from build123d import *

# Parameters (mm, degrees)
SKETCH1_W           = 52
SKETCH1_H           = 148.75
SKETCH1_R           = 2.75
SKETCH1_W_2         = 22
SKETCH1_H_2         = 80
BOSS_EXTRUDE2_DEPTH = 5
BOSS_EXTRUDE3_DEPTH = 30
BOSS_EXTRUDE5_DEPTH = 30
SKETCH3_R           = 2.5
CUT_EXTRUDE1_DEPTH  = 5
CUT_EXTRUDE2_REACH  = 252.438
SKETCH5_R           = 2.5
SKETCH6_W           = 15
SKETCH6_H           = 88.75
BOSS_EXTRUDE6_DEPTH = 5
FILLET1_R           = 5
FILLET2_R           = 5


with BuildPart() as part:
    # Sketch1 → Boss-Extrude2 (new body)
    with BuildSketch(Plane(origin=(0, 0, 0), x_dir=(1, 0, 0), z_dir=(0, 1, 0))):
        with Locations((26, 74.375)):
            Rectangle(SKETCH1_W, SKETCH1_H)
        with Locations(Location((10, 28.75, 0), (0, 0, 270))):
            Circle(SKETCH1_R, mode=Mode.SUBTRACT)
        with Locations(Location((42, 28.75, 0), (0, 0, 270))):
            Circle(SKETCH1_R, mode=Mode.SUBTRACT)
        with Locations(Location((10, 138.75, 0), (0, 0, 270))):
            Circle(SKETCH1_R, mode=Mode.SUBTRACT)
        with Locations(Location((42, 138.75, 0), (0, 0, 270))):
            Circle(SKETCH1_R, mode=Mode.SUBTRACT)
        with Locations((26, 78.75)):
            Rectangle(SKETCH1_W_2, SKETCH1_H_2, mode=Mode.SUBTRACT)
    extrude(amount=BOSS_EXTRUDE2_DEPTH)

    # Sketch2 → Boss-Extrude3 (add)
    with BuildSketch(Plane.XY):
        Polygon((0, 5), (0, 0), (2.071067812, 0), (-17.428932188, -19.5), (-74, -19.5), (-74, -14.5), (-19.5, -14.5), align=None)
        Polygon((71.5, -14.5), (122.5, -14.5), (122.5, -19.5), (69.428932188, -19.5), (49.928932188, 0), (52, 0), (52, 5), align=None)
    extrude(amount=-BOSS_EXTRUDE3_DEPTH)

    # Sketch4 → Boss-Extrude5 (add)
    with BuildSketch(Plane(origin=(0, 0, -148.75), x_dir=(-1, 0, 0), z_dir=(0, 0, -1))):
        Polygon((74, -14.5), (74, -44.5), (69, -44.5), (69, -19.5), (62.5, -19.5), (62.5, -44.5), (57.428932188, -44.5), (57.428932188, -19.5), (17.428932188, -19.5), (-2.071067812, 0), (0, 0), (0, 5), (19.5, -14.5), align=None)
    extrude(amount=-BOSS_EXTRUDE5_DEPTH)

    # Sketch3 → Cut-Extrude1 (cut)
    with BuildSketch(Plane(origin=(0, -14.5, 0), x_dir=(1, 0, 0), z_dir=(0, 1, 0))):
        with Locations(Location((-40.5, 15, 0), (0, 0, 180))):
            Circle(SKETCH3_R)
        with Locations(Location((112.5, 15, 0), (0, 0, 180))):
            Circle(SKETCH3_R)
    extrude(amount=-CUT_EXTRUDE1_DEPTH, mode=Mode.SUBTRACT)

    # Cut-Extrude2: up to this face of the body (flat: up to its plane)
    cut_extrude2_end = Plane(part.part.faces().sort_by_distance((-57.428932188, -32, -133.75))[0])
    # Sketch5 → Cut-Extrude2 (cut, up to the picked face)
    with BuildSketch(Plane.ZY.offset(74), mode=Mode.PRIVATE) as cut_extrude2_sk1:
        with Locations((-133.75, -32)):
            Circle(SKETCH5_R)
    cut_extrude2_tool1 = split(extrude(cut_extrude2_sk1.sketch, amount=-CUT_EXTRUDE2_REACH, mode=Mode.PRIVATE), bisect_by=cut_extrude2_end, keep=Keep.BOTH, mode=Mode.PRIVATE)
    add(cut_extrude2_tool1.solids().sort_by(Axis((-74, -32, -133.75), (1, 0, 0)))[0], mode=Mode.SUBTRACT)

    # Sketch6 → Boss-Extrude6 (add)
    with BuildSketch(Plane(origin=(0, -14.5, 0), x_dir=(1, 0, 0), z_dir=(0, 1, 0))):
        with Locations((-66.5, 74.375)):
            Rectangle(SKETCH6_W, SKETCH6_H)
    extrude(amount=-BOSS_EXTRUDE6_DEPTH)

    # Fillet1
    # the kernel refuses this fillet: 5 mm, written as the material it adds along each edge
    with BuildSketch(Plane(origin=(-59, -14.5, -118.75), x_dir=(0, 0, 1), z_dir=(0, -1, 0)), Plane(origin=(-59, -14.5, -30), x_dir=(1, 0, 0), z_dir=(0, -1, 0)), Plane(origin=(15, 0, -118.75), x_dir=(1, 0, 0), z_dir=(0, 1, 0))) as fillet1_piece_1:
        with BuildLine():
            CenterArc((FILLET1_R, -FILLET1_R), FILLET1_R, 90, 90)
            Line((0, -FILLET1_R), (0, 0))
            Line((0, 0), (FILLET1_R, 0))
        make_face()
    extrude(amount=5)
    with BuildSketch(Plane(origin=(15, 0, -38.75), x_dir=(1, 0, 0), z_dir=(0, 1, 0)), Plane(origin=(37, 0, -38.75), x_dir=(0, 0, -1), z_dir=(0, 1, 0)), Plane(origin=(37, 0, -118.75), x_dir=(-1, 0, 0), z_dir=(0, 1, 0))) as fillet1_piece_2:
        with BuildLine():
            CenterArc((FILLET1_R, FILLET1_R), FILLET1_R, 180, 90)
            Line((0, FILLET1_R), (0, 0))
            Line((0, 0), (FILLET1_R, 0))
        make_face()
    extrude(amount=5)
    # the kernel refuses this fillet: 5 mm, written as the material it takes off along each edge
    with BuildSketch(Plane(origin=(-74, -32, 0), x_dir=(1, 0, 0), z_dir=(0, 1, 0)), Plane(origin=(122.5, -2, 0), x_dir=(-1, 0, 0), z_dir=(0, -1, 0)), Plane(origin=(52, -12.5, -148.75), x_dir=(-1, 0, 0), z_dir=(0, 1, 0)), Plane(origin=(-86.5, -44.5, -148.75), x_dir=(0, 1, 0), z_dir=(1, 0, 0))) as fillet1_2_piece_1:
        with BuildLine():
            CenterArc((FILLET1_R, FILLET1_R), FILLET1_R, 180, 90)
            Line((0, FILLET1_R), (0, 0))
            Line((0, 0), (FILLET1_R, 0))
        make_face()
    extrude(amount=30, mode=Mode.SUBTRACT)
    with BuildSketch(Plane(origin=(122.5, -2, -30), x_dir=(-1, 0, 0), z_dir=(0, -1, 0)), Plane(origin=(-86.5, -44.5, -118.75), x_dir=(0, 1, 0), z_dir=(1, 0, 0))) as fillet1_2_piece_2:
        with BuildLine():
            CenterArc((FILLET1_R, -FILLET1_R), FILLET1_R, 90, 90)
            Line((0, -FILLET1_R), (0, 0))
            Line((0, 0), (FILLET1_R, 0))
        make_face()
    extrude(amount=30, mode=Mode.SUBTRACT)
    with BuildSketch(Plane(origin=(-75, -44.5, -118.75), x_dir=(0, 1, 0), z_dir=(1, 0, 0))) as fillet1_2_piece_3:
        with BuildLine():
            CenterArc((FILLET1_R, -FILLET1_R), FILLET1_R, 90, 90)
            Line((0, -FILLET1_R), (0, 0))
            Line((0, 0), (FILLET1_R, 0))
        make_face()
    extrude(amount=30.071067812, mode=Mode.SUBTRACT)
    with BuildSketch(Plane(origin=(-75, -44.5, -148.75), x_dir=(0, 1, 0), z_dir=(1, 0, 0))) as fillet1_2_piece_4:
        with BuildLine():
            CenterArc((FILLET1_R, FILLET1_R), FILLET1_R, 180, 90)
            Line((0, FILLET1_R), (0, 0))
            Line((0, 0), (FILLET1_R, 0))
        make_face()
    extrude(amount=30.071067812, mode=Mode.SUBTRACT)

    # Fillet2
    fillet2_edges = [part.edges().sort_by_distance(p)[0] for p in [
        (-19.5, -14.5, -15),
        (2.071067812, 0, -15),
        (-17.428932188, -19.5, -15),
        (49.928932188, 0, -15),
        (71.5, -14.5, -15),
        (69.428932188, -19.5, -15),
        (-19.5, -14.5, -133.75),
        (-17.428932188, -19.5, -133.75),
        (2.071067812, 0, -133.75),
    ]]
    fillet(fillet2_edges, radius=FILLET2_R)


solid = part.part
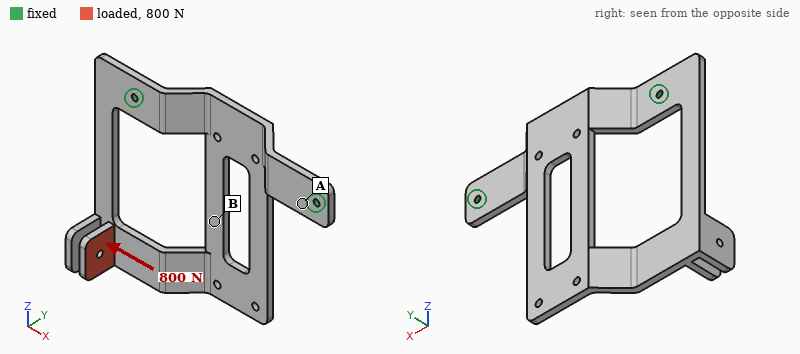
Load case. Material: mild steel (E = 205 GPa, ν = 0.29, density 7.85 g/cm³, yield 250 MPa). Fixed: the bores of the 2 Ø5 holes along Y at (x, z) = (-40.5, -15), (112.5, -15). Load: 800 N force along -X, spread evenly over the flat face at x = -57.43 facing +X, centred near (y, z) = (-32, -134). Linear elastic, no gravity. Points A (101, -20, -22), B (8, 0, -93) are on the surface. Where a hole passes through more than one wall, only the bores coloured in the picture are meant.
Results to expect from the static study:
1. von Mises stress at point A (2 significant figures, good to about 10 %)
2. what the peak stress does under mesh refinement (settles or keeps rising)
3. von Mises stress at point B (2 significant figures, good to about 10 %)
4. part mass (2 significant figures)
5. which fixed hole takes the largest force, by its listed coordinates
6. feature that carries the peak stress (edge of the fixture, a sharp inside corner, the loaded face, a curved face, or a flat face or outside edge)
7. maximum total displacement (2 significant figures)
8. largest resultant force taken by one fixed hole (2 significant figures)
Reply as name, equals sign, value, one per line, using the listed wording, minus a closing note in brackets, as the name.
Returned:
von Mises stress at point A = 31 MPa
what the peak stress does under mesh refinement = keeps rising
von Mises stress at point B = 65 MPa
part mass = 630 g
which fixed hole takes the largest force, by its listed coordinates = (-40.5, -15)
feature that carries the peak stress = edge of the fixture
maximum total displacement = 1.4 mm
largest resultant force taken by one fixed hole = 890 N
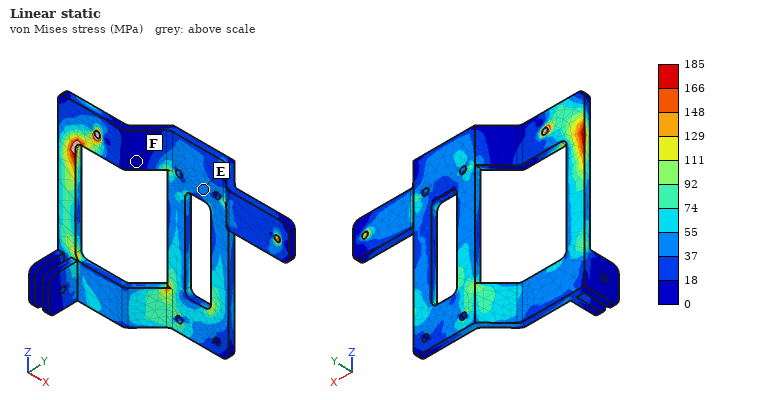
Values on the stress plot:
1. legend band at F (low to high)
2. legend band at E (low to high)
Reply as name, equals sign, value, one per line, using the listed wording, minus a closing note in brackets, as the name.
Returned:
legend band at F = 0 to 18 MPa
legend band at E = 37 to 55 MPa
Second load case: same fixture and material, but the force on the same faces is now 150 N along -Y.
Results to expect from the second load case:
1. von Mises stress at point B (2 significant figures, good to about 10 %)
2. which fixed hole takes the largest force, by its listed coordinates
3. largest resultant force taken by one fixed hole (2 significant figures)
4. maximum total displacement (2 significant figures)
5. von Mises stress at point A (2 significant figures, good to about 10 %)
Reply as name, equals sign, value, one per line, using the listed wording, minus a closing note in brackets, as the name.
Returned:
von Mises stress at point B = 22 MPa
which fixed hole takes the largest force, by its listed coordinates = (-40.5, -15)
largest resultant force taken by one fixed hole = 160 N
maximum total displacement = 1.1 mm
von Mises stress at point A = 22 MPa
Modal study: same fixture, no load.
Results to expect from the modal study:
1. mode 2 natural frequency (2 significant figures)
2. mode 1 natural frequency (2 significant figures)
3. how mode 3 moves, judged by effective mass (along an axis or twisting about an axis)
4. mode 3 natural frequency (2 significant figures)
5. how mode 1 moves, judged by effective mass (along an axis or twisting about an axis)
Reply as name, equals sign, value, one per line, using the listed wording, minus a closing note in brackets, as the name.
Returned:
mode 2 natural frequency = 330 Hz
mode 1 natural frequency = 140 Hz
how mode 3 moves, judged by effective mass = along X
mode 3 natural frequency = 650 Hz
how mode 1 moves, judged by effective mass = along Y
